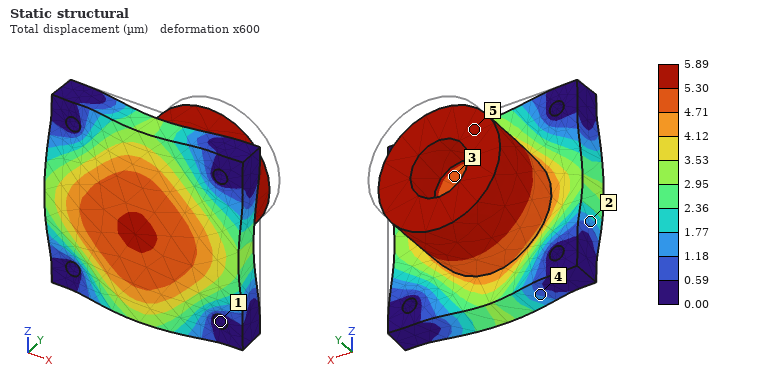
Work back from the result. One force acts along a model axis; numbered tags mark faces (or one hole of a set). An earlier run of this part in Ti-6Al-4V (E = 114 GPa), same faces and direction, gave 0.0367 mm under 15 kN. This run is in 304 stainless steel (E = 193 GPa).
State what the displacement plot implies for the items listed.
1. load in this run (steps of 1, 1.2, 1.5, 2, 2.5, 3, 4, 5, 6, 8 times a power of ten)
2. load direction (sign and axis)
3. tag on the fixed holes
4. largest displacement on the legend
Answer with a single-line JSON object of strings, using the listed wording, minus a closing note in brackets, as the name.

{"load in this run": "4 kN", "load direction": "-Y", "tag on the fixed holes": "1", "largest displacement on the legend": "5.89 µm"}
